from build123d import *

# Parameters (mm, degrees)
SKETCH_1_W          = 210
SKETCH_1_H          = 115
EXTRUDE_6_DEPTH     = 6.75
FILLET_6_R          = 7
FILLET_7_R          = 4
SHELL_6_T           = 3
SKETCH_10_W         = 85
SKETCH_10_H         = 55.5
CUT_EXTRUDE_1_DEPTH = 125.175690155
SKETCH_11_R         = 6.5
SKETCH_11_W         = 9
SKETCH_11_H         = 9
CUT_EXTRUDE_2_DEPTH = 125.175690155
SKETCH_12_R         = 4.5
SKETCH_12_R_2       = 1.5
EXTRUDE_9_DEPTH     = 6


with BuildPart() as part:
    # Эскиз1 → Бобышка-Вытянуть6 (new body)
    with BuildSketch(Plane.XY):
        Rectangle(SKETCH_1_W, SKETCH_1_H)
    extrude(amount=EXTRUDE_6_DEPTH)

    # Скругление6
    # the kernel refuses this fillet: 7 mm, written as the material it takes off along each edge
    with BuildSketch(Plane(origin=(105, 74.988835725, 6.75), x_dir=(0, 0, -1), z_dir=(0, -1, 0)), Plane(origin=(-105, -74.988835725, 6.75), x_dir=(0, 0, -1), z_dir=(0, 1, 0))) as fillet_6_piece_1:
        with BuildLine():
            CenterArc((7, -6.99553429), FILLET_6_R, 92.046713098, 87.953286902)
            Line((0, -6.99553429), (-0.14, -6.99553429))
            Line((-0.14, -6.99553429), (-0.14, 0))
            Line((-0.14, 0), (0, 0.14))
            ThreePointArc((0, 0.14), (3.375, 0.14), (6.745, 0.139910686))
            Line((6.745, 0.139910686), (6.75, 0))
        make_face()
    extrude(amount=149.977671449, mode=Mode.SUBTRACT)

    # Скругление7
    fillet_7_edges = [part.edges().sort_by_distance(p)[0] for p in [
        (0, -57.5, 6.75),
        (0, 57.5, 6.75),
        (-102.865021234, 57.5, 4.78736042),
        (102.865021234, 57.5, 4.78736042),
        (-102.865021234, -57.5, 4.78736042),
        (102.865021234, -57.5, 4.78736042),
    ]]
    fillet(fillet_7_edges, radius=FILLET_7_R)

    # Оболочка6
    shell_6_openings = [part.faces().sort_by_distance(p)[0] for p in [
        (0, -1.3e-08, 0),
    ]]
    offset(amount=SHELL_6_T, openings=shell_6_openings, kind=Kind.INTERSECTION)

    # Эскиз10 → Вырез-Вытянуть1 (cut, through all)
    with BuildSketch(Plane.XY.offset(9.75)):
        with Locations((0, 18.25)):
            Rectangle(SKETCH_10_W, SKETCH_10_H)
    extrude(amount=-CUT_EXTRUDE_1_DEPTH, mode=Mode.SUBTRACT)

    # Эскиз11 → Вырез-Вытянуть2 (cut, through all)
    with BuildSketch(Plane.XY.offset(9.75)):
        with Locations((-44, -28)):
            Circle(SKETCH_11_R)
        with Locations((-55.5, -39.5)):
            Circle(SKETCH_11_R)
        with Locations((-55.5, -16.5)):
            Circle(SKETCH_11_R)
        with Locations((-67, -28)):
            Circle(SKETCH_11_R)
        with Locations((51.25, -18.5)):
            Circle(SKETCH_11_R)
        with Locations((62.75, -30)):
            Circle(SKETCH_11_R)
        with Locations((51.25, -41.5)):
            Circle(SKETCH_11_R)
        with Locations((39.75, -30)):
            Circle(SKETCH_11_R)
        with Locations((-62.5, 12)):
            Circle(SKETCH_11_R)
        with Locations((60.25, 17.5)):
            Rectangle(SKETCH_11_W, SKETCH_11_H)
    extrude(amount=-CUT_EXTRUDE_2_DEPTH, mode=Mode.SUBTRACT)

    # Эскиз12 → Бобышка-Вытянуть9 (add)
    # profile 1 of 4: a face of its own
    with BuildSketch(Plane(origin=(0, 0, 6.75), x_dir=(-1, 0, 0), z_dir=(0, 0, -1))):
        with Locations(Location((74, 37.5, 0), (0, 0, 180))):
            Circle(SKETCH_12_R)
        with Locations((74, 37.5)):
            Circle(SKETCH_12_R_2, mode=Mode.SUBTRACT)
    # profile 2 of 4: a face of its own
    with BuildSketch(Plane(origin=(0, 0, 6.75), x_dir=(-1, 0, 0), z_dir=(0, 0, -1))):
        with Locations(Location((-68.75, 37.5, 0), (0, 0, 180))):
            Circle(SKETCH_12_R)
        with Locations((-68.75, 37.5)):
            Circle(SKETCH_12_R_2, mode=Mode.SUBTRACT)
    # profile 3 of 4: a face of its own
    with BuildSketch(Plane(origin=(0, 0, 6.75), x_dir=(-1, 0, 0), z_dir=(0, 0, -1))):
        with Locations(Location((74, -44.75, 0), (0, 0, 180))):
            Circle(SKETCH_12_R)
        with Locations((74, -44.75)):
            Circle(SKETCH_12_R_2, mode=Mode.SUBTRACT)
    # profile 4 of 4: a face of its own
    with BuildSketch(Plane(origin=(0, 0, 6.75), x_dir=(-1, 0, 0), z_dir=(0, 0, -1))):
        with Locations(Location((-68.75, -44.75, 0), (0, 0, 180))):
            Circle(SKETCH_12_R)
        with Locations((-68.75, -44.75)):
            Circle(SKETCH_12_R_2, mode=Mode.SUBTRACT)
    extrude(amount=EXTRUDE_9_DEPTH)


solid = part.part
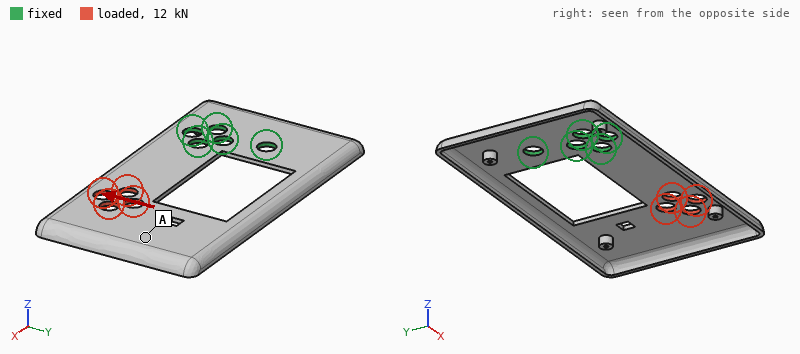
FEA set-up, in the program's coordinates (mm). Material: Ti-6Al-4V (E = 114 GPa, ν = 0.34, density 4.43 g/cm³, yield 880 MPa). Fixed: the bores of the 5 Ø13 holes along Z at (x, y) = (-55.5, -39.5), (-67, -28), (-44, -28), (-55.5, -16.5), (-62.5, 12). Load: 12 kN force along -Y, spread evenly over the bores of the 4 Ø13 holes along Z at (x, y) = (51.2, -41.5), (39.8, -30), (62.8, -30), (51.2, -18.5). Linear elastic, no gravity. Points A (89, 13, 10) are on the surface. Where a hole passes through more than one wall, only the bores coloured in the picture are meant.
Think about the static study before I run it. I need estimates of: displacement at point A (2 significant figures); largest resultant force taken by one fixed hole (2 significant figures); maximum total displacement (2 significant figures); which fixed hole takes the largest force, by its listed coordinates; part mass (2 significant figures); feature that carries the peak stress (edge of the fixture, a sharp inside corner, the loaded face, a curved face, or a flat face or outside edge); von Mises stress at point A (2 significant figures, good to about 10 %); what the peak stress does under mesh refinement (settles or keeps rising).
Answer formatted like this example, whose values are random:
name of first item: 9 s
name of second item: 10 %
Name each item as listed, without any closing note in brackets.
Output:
displacement at point A: 0.98 mm
largest resultant force taken by one fixed hole: 21 kN
maximum total displacement: 2.1 mm
which fixed hole takes the largest force, by its listed coordinates: (-55.5, -39.5)
part mass: 310 g
feature that carries the peak stress: a sharp inside corner
von Mises stress at point A: 66 MPa
what the peak stress does under mesh refinement: keeps rising
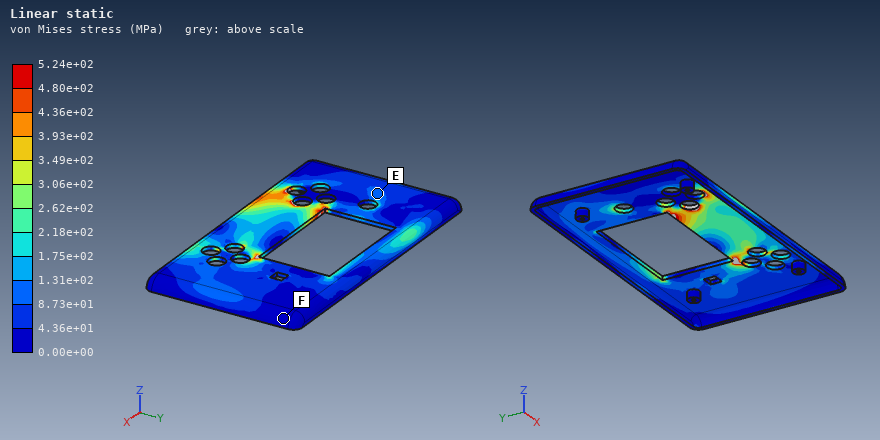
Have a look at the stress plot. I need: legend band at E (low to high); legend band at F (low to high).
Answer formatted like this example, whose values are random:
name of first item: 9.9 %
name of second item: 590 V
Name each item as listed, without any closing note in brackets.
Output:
legend band at E: 8.73e+01 to 1.31e+02 MPa
legend band at F: 0.00e+00 to 4.36e+01 MPa
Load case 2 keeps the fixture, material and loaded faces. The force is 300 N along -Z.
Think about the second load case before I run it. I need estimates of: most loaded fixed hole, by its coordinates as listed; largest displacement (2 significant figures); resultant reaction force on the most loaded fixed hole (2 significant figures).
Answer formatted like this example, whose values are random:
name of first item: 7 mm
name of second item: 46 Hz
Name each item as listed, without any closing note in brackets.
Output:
most loaded fixed hole, by its coordinates as listed: (-44, -28)
largest displacement: 2.7 mm
resultant reaction force on the most loaded fixed hole: 980 N
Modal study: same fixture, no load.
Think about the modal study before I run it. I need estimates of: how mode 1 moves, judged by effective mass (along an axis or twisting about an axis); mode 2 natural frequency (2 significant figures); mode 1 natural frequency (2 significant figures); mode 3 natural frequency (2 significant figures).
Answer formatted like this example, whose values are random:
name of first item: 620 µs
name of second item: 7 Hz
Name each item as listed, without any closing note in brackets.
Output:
how mode 1 moves, judged by effective mass: along Z
mode 2 natural frequency: 280 Hz
mode 1 natural frequency: 130 Hz
mode 3 natural frequency: 830 Hz
